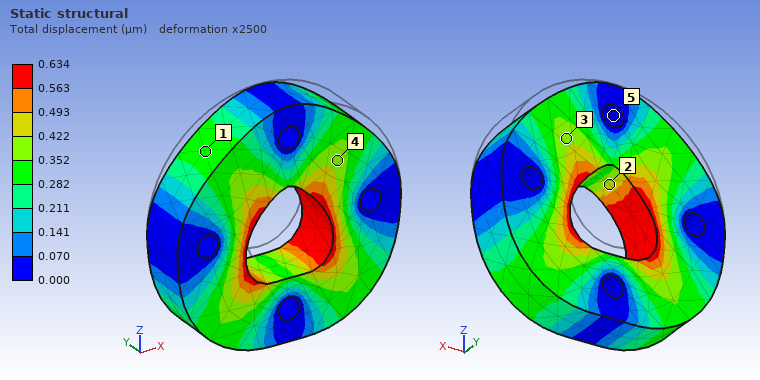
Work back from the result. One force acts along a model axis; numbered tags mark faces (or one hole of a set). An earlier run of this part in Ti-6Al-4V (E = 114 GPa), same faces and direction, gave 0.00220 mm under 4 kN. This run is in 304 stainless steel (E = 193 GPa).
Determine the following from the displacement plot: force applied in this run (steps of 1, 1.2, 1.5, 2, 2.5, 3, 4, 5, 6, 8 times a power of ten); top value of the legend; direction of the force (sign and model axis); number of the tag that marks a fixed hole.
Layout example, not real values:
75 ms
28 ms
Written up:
2 kN
0.634 µm
-Z
5
